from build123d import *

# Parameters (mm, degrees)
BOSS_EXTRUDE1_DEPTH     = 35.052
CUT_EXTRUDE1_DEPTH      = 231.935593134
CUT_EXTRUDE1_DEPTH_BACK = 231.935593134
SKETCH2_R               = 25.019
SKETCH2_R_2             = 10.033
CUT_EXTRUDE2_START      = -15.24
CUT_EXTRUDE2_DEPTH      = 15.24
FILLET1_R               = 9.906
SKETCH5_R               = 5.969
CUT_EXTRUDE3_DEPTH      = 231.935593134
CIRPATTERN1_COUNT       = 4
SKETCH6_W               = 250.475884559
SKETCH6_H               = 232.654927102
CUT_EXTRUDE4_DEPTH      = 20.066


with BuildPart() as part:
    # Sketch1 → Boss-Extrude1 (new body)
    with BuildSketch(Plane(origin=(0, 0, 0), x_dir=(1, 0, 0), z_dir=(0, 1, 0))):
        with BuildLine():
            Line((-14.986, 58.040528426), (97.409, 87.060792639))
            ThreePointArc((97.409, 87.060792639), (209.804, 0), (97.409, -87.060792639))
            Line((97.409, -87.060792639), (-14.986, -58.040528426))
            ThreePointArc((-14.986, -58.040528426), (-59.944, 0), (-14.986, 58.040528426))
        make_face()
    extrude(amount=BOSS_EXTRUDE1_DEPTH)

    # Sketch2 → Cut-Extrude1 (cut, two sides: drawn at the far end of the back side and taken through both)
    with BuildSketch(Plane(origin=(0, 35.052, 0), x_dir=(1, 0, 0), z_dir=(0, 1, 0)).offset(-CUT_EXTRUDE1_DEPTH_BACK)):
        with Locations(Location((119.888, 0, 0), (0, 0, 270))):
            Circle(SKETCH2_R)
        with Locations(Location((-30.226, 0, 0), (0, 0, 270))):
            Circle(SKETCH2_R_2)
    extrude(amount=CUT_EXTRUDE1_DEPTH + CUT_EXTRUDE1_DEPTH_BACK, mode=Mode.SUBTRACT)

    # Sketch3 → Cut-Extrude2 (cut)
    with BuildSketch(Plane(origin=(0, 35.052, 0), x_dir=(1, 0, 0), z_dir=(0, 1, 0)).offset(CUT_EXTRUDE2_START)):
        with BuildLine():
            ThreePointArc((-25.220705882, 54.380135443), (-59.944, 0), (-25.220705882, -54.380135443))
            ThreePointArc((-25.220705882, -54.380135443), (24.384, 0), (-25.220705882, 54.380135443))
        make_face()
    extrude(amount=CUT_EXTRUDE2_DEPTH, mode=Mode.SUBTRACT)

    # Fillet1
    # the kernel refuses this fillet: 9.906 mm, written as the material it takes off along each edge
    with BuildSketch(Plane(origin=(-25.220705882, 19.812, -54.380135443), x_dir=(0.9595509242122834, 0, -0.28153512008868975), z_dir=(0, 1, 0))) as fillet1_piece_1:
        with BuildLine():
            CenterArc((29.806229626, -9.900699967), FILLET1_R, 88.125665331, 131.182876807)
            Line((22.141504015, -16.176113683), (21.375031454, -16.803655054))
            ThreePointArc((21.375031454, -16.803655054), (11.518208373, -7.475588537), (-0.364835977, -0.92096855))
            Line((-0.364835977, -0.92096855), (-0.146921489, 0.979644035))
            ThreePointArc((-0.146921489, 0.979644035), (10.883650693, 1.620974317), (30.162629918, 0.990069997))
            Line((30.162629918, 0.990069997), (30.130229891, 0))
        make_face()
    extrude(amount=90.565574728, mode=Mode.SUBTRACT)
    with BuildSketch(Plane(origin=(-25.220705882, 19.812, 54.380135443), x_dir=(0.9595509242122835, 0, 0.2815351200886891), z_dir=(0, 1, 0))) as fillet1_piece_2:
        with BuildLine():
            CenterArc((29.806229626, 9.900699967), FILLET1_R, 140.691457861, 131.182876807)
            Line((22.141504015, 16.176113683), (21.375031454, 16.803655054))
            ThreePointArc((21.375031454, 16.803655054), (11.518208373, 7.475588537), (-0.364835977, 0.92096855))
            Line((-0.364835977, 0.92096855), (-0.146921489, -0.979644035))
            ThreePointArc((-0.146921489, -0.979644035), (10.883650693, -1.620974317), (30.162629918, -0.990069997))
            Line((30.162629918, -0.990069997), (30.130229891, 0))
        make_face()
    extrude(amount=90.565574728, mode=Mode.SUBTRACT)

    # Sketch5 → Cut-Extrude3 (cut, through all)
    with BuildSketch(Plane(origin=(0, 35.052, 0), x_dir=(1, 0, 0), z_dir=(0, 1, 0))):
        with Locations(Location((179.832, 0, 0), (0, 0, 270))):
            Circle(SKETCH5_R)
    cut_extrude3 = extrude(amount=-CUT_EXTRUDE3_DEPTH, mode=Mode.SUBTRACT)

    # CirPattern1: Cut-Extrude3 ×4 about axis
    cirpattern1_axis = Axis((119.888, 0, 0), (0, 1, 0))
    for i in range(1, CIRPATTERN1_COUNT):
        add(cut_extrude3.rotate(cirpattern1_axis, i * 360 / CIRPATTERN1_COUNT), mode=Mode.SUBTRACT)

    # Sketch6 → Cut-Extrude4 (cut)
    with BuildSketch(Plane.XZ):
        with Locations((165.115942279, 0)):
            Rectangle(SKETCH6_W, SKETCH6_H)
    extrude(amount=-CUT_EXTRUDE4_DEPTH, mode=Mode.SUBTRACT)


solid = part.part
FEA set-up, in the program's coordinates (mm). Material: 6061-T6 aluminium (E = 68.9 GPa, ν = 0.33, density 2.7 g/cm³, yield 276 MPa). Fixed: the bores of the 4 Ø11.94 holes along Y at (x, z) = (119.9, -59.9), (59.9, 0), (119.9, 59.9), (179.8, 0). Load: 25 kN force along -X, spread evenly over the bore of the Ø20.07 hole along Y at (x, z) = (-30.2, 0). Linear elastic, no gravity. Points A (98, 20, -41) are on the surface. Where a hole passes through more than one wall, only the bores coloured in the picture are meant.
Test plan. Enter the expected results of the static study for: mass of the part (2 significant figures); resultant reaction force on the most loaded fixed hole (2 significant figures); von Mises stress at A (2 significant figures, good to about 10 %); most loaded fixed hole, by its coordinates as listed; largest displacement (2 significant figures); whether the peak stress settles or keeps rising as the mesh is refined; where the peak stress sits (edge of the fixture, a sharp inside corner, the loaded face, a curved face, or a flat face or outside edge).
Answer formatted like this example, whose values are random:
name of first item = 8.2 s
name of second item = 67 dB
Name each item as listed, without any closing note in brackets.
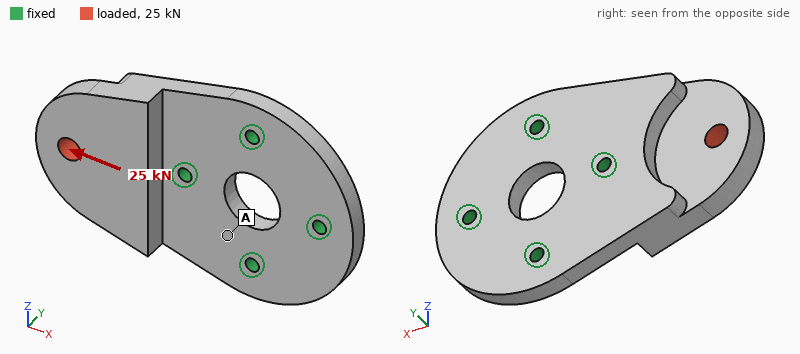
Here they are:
mass of the part = 1.7 kg
resultant reaction force on the most loaded fixed hole = 14 kN
von Mises stress at A = 14 MPa
most loaded fixed hole, by its coordinates as listed = (59.9, 0)
largest displacement = 0.59 mm
whether the peak stress settles or keeps rising as the mesh is refined = keeps rising
where the peak stress sits = edge of the fixture
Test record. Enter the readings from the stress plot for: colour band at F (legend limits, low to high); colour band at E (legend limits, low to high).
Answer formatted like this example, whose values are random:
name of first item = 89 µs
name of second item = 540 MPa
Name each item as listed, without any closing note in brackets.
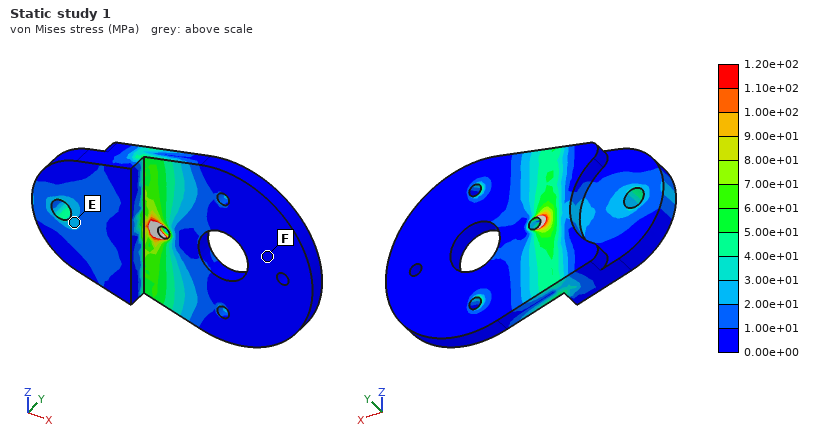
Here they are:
colour band at F = 0.00e+00 to 1.00e+01 MPa
colour band at E = 2.00e+01 to 3.00e+01 MPa
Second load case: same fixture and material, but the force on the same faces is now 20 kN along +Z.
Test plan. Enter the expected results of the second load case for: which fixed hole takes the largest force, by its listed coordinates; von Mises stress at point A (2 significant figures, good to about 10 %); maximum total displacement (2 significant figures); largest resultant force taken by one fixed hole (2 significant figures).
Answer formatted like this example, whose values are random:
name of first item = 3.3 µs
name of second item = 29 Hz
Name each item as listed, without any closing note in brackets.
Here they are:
which fixed hole takes the largest force, by its listed coordinates = (59.9, 0)
von Mises stress at point A = 13 MPa
maximum total displacement = 0.14 mm
largest resultant force taken by one fixed hole = 20 kN
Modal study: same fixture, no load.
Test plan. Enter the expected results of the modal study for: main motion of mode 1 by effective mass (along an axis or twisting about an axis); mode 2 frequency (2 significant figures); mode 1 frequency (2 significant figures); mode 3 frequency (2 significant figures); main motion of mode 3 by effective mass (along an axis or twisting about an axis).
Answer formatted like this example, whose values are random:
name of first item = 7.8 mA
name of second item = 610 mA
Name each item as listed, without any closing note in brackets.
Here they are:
main motion of mode 1 by effective mass = along Y
mode 2 frequency = 1700 Hz
mode 1 frequency = 920 Hz
mode 3 frequency = 3400 Hz
main motion of mode 3 by effective mass = along Z
